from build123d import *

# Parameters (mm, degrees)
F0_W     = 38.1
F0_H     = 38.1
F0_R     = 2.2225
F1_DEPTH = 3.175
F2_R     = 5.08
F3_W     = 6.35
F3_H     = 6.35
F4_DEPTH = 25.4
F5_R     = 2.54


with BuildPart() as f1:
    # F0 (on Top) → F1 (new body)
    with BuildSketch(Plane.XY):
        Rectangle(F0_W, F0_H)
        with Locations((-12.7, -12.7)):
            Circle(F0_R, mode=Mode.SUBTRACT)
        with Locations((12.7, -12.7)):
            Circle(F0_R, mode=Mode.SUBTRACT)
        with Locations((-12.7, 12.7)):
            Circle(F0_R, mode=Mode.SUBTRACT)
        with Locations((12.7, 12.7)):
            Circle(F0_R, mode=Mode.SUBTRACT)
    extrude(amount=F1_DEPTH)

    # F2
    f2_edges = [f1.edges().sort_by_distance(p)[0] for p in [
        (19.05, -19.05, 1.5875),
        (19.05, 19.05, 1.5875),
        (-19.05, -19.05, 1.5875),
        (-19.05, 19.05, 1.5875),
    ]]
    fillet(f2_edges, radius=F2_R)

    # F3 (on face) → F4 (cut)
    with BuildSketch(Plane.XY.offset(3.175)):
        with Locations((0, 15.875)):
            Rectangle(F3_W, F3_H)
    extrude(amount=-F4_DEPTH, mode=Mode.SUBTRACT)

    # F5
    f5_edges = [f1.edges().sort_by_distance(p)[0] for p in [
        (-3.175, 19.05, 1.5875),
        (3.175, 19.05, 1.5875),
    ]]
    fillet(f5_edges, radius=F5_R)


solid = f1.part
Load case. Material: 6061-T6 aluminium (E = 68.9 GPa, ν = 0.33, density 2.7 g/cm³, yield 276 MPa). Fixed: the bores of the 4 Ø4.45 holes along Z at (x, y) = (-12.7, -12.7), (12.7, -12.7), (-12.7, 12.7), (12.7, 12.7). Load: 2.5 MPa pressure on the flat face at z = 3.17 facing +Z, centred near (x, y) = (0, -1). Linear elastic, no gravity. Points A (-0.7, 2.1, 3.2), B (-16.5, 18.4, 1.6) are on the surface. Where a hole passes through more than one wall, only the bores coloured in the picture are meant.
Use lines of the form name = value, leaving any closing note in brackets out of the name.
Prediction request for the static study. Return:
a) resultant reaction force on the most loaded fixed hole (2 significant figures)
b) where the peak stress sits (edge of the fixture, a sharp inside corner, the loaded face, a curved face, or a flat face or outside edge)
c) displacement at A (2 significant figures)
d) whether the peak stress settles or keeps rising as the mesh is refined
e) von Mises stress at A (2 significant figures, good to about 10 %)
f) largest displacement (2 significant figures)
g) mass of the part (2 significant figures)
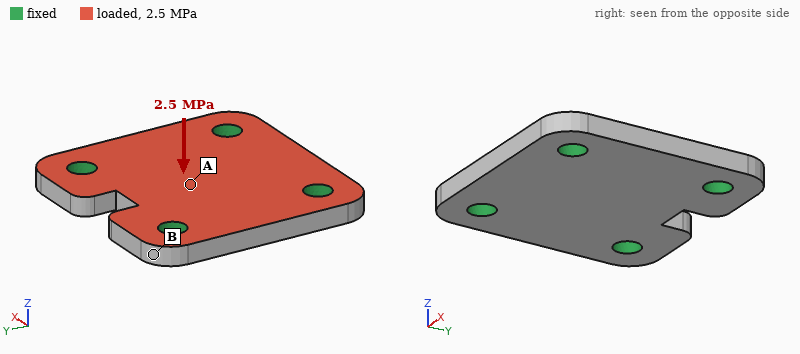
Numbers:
resultant reaction force on the most loaded fixed hole = 860 N
where the peak stress sits = edge of the fixture
displacement at A = 26 µm
whether the peak stress settles or keeps rising as the mesh is refined = keeps rising
von Mises stress at A = 35 MPa
largest displacement = 26 µm
mass of the part = 11 g
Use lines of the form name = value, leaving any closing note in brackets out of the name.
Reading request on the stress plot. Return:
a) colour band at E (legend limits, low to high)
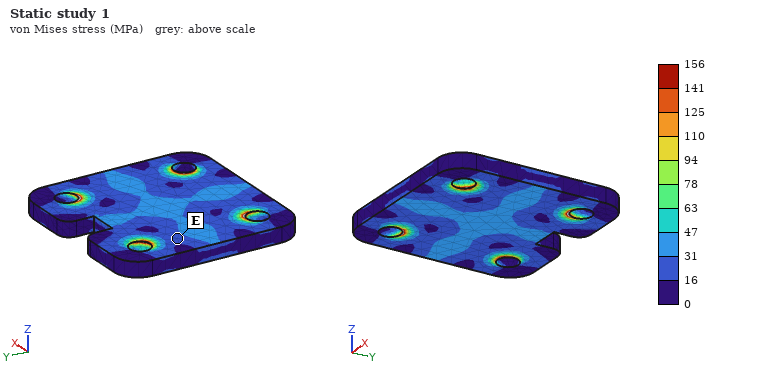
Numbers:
colour band at E = 16 to 31 MPa
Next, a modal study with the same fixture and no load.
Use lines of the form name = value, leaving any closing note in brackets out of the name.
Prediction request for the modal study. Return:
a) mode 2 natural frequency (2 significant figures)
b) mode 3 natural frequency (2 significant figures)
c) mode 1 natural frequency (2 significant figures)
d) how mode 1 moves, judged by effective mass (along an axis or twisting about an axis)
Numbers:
mode 2 natural frequency = 28 kHz
mode 3 natural frequency = 28 kHz
mode 1 natural frequency = 20 kHz
how mode 1 moves, judged by effective mass = along Z
